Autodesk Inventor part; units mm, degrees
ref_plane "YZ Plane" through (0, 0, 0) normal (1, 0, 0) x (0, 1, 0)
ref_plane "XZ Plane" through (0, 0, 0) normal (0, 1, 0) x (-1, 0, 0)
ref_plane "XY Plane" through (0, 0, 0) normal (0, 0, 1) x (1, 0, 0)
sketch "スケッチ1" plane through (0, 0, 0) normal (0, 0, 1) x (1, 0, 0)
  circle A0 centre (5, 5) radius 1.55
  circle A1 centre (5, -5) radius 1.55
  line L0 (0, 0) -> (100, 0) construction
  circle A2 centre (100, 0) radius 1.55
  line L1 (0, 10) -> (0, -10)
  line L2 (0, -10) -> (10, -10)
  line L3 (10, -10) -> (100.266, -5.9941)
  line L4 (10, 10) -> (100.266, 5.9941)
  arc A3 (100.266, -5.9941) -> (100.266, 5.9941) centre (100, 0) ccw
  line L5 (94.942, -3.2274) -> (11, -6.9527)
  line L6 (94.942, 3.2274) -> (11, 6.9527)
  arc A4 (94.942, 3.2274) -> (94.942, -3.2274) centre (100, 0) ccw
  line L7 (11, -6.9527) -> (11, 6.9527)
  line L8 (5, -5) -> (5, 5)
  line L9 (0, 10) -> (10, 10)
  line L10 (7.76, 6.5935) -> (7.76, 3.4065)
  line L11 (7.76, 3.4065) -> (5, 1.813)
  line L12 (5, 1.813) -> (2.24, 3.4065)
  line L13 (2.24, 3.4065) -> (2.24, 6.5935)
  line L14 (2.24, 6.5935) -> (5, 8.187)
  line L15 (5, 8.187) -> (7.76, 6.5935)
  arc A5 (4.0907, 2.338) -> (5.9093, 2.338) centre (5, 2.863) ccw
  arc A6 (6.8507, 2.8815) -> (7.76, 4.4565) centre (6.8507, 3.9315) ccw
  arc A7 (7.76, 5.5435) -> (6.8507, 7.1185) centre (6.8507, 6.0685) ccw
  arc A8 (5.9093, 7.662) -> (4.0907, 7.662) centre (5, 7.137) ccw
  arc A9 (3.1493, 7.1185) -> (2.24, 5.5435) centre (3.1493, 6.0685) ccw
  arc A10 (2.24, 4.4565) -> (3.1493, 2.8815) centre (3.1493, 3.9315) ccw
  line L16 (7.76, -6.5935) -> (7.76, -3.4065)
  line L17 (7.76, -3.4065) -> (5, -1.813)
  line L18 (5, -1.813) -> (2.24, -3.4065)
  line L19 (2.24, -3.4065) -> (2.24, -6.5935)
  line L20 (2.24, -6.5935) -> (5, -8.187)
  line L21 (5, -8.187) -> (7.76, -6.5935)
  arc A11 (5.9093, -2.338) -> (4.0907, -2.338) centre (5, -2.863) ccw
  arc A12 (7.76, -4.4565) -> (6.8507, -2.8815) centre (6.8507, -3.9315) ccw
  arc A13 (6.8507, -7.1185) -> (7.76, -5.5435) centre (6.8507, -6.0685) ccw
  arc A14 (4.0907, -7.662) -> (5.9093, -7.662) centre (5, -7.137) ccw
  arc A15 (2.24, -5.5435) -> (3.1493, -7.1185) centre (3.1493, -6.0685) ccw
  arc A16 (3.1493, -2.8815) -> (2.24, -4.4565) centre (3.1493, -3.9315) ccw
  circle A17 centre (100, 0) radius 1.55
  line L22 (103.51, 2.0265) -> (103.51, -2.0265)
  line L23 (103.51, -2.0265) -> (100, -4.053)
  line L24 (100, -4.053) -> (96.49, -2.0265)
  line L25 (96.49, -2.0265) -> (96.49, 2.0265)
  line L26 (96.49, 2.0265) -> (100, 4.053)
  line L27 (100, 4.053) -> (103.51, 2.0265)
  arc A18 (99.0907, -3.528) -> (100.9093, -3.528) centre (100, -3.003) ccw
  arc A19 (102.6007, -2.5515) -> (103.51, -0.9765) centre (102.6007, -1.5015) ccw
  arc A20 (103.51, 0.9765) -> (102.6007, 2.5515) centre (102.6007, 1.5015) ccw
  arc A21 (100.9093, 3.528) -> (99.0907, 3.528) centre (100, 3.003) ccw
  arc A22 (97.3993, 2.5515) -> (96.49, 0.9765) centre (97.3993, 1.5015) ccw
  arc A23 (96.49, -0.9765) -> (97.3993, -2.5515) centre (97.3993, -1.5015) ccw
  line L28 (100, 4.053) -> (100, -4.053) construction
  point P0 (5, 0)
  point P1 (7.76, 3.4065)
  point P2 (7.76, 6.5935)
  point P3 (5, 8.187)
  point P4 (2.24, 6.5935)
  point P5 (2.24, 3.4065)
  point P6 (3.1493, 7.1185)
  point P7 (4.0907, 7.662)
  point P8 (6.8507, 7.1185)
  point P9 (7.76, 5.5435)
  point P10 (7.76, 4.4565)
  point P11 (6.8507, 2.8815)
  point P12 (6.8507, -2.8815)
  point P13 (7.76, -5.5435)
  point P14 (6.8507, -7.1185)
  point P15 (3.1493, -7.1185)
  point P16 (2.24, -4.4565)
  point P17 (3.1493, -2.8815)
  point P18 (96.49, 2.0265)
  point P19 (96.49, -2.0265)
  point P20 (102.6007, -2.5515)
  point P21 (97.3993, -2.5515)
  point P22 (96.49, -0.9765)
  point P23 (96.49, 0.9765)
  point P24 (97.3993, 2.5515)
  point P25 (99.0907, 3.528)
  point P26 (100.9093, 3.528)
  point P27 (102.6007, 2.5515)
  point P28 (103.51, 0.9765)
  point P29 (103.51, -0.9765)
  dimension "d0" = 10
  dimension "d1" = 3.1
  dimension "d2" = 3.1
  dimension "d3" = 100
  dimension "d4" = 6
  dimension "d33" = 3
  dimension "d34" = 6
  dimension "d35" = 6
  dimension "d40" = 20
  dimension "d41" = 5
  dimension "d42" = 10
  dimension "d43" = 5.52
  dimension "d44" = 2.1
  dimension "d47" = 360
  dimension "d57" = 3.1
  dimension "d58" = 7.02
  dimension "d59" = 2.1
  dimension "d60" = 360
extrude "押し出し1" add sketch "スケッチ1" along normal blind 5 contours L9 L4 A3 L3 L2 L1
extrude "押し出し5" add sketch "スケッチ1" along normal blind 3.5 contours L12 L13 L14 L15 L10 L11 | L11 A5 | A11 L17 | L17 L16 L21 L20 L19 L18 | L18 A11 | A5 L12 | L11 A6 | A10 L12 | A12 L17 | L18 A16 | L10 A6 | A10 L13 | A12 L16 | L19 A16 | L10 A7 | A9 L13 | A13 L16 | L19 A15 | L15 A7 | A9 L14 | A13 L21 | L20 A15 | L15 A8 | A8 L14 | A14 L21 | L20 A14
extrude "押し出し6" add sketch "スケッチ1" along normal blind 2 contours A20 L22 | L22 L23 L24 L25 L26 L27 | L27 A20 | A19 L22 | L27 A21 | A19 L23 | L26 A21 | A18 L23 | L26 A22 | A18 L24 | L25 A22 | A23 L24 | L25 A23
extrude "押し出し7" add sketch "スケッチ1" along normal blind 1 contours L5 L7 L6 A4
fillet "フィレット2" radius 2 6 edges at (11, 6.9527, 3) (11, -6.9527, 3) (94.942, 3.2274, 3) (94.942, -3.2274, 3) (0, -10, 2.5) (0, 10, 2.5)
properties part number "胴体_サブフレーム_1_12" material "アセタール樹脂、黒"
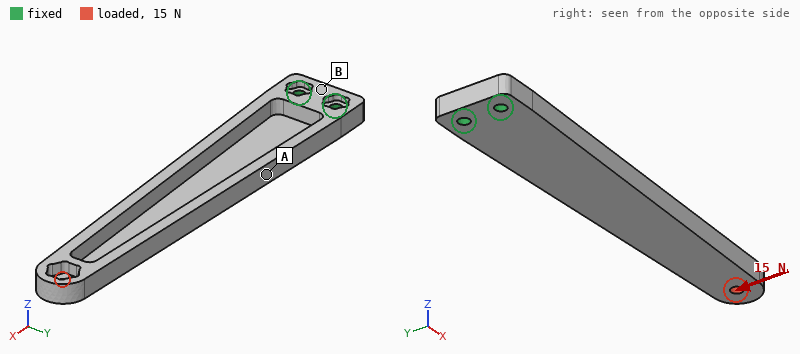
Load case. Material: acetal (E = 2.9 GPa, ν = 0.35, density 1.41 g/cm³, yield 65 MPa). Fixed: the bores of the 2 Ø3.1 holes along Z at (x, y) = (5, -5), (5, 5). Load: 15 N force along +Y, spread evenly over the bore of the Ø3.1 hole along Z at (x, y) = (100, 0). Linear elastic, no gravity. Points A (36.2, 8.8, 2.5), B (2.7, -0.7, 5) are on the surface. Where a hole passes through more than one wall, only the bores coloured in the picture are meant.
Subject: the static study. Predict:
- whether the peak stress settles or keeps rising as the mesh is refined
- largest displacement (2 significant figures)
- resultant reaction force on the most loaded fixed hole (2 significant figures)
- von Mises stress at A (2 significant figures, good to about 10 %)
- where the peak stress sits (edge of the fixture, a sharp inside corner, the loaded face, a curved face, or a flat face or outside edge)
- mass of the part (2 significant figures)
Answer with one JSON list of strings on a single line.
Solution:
["keeps rising", "1.0 mm", "120 N", "4.9 MPa", "edge of the fixture", "6.8 g"]
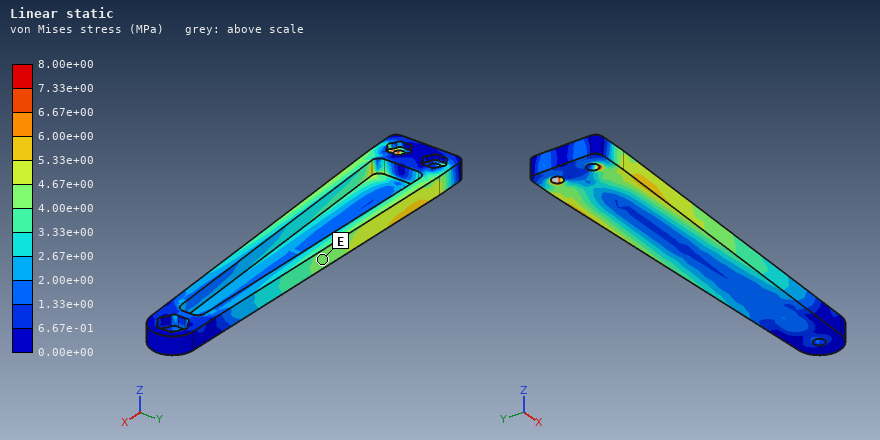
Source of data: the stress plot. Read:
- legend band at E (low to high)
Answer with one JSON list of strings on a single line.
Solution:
["4.00e+00 to 4.67e+00 MPa"]
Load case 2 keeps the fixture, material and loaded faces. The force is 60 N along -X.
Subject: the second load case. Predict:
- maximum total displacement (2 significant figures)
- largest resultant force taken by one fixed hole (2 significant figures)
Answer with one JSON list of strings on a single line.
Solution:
["1.0 mm", "30 N"]
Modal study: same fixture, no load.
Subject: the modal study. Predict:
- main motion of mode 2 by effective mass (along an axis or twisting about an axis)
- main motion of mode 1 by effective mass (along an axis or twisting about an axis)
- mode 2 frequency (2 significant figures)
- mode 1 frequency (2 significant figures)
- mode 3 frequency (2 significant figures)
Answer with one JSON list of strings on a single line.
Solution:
["along Y", "along Z", "460 Hz", "130 Hz", "710 Hz"]
